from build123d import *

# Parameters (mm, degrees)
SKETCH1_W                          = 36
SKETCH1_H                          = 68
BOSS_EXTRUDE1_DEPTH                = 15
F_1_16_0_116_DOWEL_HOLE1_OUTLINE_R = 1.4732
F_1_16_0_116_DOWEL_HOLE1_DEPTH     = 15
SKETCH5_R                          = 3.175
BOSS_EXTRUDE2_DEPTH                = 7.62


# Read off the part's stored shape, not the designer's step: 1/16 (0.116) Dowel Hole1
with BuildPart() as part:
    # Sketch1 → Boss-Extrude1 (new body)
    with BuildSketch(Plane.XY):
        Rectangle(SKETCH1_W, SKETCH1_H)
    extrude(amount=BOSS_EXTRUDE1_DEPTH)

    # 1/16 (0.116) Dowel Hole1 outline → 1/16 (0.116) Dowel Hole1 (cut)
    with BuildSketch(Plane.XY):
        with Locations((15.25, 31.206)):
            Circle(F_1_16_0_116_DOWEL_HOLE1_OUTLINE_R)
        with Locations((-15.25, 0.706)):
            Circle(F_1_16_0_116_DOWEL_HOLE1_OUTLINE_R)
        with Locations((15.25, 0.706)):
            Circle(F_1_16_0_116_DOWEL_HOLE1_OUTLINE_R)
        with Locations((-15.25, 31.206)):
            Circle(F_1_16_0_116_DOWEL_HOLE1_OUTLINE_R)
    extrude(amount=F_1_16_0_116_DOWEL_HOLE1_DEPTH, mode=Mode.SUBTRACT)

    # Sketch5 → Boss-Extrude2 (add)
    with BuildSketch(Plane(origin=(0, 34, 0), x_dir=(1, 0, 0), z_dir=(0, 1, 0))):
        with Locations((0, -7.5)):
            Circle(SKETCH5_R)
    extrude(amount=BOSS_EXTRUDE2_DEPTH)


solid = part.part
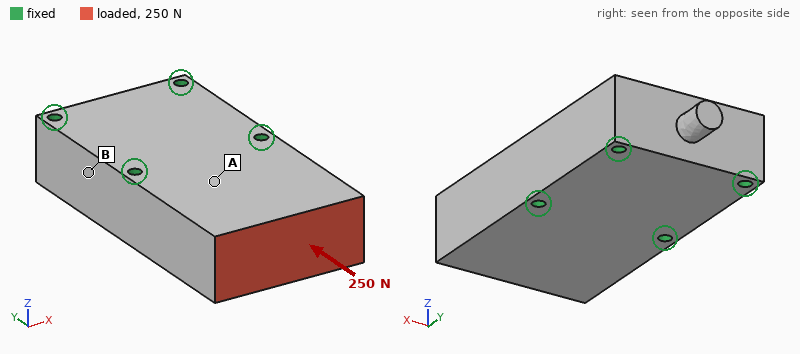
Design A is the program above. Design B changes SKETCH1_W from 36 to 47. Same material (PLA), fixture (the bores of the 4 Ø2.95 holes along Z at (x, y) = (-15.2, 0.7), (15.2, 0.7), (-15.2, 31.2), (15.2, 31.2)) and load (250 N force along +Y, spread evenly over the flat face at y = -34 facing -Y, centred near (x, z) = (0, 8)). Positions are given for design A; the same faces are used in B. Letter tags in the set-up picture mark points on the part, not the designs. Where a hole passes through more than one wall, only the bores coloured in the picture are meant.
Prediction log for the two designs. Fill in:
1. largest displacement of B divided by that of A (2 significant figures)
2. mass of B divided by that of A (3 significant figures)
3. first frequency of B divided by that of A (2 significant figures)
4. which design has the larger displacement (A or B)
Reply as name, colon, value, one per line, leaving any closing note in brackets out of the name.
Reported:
largest displacement of B divided by that of A: 0.79
mass of B divided by that of A: 1.31
first frequency of B divided by that of A: 1.00
which design has the larger displacement: A
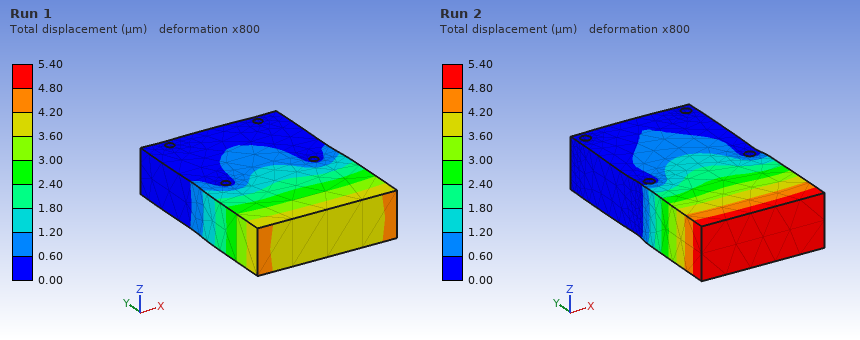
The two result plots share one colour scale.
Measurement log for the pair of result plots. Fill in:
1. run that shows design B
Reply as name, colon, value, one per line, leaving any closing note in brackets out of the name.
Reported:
run that shows design B: Run 1
